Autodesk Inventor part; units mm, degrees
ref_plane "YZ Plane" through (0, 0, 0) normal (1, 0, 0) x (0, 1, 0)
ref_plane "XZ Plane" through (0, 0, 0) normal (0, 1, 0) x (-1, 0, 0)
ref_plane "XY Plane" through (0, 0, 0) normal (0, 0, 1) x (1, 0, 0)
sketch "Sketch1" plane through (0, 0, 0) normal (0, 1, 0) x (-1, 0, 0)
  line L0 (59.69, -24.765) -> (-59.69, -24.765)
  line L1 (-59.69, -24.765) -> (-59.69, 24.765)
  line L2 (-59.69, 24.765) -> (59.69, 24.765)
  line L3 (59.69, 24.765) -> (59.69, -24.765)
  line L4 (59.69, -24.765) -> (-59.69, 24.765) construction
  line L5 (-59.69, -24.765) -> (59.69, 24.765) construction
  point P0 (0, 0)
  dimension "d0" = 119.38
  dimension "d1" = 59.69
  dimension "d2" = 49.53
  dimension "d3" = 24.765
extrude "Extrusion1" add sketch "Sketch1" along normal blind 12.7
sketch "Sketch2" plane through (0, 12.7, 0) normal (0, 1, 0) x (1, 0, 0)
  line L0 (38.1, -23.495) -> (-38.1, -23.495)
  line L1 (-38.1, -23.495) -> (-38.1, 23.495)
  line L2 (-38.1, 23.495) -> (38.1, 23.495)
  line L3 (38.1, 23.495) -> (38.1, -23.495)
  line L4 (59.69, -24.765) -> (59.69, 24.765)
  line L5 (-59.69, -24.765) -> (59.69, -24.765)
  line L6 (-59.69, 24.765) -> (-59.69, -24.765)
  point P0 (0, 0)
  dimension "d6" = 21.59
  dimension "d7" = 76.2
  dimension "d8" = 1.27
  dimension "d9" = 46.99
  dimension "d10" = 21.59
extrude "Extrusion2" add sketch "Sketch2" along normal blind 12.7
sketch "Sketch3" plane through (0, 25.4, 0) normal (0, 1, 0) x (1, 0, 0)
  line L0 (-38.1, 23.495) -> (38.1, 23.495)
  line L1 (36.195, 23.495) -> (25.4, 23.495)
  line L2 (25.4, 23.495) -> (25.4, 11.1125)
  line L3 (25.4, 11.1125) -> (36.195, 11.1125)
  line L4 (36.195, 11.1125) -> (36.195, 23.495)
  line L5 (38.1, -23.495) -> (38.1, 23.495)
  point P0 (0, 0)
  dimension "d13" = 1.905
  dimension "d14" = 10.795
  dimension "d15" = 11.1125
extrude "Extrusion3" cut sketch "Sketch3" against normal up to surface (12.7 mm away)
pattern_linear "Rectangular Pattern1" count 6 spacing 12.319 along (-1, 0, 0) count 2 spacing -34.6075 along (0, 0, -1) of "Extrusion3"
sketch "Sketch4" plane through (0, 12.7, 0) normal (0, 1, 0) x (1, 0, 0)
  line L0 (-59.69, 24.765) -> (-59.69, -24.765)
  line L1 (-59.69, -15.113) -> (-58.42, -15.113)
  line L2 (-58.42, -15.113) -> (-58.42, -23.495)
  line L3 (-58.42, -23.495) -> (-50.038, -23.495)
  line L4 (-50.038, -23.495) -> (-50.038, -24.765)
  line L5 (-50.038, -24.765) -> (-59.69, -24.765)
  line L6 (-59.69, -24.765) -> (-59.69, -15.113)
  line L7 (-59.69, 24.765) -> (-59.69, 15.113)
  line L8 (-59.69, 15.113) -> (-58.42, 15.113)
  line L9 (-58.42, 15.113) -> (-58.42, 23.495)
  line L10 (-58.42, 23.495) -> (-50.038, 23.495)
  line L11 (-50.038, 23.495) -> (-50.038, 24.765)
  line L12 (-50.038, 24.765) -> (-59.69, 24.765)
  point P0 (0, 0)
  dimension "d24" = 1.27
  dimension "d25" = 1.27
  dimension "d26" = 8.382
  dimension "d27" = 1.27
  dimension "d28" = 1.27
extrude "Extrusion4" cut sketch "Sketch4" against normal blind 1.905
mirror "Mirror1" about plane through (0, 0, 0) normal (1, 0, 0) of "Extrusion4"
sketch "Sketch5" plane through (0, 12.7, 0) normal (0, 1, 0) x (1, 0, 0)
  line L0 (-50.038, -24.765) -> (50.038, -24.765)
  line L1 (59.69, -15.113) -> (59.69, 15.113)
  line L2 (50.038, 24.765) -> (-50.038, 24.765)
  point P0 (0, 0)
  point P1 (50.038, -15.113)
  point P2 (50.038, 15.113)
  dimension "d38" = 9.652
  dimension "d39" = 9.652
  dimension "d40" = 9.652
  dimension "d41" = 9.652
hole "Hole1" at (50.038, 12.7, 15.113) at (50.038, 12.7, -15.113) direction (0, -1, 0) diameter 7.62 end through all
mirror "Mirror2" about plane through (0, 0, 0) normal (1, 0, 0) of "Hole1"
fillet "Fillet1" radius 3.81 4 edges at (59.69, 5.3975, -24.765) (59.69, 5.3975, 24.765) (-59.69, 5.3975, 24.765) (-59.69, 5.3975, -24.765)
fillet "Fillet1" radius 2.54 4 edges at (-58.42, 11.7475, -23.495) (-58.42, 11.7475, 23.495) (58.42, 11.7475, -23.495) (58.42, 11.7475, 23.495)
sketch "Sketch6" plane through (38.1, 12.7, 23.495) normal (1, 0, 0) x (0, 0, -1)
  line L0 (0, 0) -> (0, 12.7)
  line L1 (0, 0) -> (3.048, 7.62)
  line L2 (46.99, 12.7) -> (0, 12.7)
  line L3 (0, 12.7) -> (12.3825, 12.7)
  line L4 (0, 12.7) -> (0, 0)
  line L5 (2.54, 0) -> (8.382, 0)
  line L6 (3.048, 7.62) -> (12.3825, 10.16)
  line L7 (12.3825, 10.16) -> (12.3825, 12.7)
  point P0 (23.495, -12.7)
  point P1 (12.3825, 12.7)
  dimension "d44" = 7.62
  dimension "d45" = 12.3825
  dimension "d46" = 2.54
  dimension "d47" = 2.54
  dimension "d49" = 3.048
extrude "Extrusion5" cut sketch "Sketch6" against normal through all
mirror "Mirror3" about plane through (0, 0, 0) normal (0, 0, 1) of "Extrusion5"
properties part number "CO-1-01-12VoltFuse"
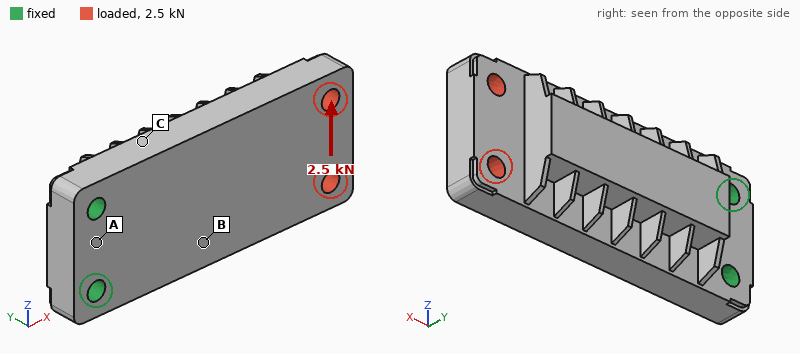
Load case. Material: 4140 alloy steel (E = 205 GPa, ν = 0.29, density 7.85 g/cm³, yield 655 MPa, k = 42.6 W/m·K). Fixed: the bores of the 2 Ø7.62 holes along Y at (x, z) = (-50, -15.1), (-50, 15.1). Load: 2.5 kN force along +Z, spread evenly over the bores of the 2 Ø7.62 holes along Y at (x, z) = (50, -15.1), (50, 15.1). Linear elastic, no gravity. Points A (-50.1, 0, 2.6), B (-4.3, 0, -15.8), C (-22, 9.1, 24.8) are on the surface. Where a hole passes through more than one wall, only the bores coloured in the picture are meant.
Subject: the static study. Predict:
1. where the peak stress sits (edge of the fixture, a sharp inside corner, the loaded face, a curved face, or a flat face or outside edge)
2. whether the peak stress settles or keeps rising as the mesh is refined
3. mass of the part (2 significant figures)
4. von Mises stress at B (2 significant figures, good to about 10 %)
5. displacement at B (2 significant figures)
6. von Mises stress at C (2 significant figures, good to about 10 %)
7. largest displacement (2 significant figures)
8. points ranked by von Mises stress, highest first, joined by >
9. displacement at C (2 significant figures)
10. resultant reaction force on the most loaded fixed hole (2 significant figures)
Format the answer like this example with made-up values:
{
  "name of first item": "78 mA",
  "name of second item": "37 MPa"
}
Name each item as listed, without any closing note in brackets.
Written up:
{
  "where the peak stress sits": "edge of the fixture",
  "whether the peak stress settles or keeps rising as the mesh is refined": "keeps rising",
  "mass of the part": "750 g",
  "von Mises stress at B": "17 MPa",
  "displacement at B": "12 µm",
  "von Mises stress at C": "33 MPa",
  "largest displacement": "43 µm",
  "points ranked by von Mises stress, highest first, joined by >": "C > B > A",
  "displacement at C": "8.0 µm",
  "resultant reaction force on the most loaded fixed hole": "7.4 kN"
}
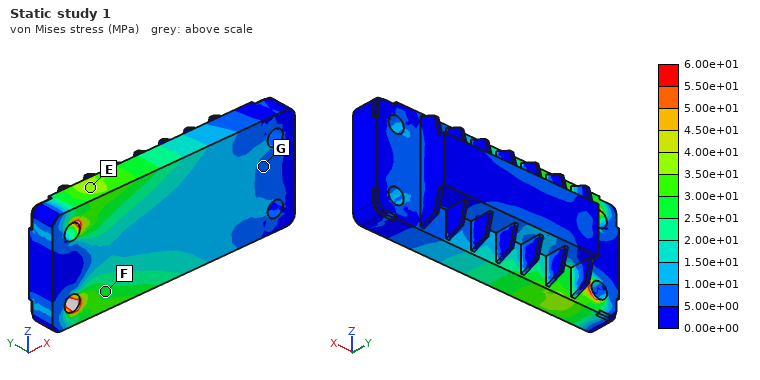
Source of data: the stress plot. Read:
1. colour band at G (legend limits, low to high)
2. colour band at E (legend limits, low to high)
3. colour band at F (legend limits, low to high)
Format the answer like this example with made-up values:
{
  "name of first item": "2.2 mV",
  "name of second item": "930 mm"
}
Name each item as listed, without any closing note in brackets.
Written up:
{
  "colour band at G": "5.00e+00 to 1.00e+01 MPa",
  "colour band at E": "3.50e+01 to 4.00e+01 MPa",
  "colour band at F": "2.50e+01 to 3.00e+01 MPa"
}
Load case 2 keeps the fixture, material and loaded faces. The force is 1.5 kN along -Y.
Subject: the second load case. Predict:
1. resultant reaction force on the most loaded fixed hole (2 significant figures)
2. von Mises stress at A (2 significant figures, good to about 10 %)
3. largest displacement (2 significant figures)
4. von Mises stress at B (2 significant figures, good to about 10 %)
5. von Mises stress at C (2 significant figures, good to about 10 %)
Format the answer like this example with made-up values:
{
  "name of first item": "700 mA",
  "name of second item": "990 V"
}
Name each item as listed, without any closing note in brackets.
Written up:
{
  "resultant reaction force on the most loaded fixed hole": "840 N",
  "von Mises stress at A": "36 MPa",
  "largest displacement": "0.19 mm",
  "von Mises stress at B": "20 MPa",
  "von Mises stress at C": "17 MPa"
}
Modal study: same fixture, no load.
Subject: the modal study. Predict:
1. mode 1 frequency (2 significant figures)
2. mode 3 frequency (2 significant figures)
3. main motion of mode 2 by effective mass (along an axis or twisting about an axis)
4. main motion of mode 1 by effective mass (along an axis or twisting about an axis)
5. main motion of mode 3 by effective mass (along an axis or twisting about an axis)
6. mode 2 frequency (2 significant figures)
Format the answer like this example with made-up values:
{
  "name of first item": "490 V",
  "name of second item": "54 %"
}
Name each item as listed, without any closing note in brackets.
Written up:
{
  "mode 1 frequency": "990 Hz",
  "mode 3 frequency": "4700 Hz",
  "main motion of mode 2 by effective mass": "along Z",
  "main motion of mode 1 by effective mass": "along Y",
  "main motion of mode 3 by effective mass": "twisting about X",
  "mode 2 frequency": "2800 Hz"
}
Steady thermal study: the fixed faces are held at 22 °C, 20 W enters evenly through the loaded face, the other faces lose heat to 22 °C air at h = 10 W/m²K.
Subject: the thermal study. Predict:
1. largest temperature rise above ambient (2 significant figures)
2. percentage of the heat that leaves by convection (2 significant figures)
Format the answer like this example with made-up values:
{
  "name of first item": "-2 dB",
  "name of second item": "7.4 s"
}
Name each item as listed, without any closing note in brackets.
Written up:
{
  "largest temperature rise above ambient": "54 K",
  "percentage of the heat that leaves by convection": "25 %"
}
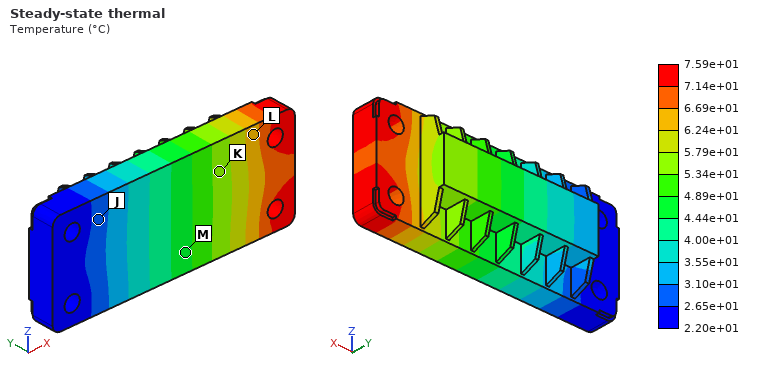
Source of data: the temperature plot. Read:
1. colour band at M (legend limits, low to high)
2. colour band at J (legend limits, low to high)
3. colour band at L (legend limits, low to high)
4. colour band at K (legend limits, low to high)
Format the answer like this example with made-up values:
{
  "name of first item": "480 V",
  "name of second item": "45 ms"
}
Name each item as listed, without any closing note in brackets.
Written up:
{
  "colour band at M": "4.44e+01 to 4.89e+01 °C",
  "colour band at J": "2.65e+01 to 3.10e+01 °C",
  "colour band at L": "6.24e+01 to 6.69e+01 °C",
  "colour band at K": "5.34e+01 to 5.79e+01 °C"
}
